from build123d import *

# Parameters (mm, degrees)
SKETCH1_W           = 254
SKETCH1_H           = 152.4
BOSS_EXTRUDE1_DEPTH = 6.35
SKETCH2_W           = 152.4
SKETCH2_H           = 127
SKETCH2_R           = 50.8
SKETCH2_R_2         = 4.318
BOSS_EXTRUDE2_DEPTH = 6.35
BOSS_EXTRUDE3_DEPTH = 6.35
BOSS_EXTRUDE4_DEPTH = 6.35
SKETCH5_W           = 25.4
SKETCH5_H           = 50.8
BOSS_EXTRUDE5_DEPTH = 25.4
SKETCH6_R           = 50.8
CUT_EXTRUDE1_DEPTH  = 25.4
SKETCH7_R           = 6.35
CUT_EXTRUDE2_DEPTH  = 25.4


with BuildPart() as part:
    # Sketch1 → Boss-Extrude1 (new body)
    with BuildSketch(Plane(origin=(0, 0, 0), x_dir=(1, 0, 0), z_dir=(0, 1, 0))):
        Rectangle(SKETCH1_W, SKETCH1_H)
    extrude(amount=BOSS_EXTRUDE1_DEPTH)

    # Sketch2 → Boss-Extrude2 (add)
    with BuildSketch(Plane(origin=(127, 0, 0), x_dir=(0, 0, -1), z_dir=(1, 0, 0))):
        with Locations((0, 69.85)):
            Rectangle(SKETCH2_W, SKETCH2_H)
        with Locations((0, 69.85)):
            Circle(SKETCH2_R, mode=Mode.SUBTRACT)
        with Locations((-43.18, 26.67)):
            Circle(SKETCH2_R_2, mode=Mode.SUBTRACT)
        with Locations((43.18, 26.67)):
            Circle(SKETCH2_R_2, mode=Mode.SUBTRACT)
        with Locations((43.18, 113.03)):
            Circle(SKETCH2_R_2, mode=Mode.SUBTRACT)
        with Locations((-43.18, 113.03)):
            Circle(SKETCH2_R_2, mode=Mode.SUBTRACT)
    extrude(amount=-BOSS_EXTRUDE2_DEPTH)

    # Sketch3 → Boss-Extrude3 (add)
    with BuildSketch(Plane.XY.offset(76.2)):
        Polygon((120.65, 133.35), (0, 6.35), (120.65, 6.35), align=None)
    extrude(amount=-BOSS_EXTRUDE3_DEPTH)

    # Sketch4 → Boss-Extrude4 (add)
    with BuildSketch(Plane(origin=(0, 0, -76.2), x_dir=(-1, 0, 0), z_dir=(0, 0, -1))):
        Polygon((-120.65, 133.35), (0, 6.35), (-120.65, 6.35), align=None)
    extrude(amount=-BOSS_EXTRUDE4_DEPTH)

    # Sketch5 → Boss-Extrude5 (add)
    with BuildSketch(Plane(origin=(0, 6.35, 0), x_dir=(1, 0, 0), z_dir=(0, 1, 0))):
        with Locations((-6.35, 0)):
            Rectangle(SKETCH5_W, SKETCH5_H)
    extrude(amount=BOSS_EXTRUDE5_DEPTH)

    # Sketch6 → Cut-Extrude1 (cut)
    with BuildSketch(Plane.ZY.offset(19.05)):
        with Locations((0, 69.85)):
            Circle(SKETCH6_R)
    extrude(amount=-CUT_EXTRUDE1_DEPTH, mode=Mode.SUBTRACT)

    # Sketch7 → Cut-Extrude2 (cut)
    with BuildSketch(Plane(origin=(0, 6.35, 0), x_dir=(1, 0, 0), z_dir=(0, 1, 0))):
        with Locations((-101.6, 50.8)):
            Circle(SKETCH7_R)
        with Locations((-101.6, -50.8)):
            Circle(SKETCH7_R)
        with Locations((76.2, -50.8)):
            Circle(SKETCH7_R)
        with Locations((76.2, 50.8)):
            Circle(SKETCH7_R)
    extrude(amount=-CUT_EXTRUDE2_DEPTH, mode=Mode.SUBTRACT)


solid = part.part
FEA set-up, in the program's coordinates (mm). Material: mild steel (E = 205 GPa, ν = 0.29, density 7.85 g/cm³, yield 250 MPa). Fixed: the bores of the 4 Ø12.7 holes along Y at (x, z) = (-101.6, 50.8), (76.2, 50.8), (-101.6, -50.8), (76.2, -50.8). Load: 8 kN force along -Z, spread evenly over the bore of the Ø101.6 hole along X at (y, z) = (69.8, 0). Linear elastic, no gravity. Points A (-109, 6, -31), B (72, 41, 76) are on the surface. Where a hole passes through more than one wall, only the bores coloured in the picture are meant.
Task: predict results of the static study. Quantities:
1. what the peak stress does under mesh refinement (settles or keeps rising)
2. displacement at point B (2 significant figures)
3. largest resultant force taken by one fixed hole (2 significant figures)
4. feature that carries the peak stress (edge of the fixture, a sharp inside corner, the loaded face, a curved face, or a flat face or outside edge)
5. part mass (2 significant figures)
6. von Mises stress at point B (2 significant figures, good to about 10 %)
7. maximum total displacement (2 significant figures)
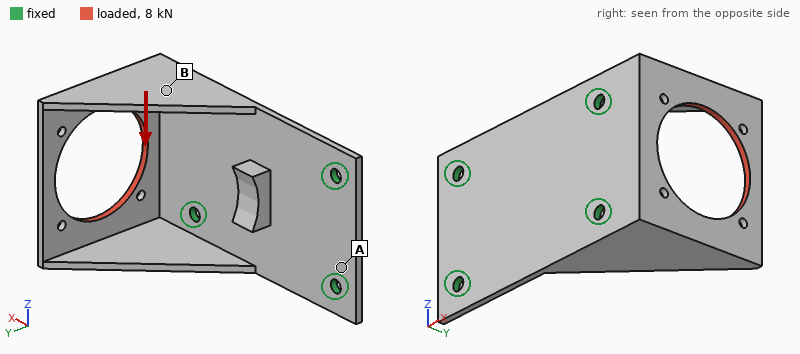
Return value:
keeps rising
0.12 mm
7.1 kN
edge of the fixture
3.4 kg
28 MPa
0.49 mm
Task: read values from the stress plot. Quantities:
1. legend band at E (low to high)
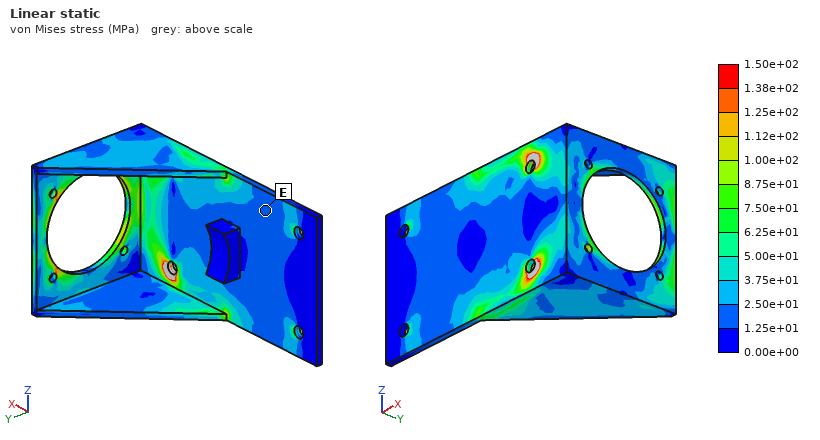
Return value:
1.25e+01 to 2.50e+01 MPa
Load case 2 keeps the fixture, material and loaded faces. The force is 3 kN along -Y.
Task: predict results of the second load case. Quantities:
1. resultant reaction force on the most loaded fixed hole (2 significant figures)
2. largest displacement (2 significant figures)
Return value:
1.8 kN
0.14 mm
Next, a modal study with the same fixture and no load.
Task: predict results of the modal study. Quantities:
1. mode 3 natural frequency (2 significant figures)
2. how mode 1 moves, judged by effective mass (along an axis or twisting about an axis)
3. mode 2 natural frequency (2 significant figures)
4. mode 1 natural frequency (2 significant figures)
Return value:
1200 Hz
along X
630 Hz
590 Hz
